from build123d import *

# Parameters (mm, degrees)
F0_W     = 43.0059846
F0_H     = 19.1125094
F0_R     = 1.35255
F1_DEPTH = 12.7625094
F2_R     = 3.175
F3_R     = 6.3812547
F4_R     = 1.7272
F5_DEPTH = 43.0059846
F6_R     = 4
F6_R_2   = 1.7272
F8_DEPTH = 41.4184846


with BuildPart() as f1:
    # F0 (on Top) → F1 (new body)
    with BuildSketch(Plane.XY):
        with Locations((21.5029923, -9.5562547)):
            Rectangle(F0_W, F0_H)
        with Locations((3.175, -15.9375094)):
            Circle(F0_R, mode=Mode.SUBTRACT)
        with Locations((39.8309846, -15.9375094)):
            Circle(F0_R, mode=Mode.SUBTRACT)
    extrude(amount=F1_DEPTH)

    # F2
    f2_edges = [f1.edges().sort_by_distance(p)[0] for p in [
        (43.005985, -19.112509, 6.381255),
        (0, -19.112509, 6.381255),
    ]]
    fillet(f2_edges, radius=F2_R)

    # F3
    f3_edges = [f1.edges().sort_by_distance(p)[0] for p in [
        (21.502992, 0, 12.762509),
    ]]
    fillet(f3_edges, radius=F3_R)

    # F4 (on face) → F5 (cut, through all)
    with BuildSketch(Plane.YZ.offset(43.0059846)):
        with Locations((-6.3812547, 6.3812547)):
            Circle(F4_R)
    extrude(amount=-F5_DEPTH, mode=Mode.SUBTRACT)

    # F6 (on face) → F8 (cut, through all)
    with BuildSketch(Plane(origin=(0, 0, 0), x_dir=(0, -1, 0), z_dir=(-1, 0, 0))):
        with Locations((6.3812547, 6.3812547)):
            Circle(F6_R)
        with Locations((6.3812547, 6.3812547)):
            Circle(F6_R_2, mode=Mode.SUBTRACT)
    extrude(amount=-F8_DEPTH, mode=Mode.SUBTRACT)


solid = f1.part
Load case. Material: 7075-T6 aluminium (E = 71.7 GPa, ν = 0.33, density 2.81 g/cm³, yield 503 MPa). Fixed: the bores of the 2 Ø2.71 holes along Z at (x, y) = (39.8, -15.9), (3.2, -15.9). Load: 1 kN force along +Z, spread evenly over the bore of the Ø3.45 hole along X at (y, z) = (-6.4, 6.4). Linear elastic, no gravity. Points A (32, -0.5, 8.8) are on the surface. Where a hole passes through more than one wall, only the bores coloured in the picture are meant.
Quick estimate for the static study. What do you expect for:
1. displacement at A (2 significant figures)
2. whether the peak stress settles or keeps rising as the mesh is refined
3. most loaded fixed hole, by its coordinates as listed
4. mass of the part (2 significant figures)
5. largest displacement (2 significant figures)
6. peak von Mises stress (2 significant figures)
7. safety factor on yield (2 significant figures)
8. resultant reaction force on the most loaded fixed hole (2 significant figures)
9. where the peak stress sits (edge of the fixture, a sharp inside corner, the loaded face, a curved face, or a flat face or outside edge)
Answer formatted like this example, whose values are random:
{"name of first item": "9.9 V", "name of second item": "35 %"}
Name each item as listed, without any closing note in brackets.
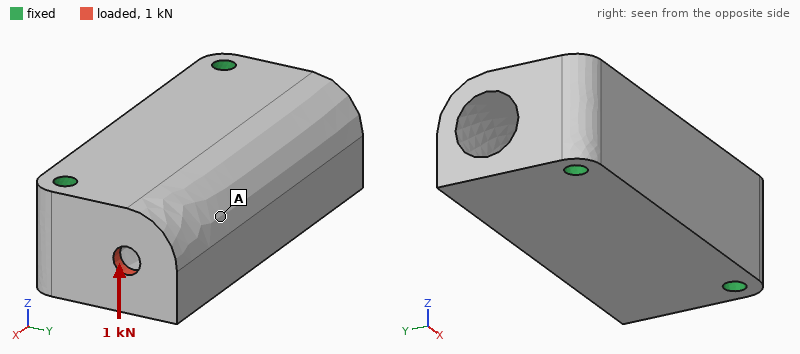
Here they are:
{"displacement at A": "7.6 µm", "whether the peak stress settles or keeps rising as the mesh is refined": "settles", "most loaded fixed hole, by its coordinates as listed": "(39.8, -15.9)", "mass of the part": "22 g", "largest displacement": "15 µm", "peak von Mises stress": "130 MPa", "safety factor on yield": "3.8", "resultant reaction force on the most loaded fixed hole": "1.0 kN", "where the peak stress sits": "the loaded face"}
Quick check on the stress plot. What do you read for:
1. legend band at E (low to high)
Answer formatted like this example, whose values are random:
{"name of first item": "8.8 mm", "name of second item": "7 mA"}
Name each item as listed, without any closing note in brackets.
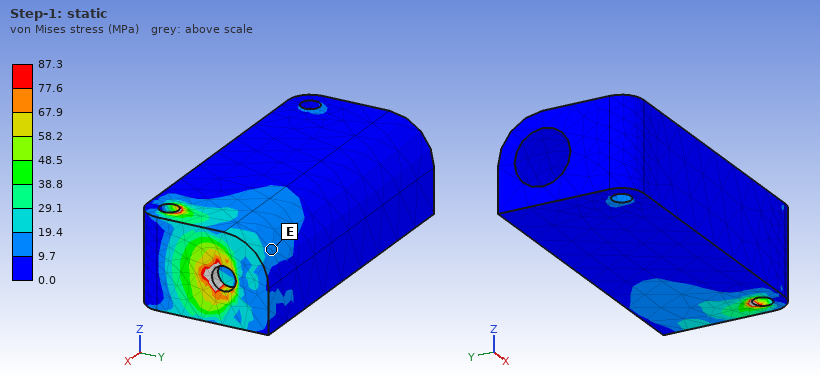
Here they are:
{"legend band at E": "9.7 to 19.4 MPa"}
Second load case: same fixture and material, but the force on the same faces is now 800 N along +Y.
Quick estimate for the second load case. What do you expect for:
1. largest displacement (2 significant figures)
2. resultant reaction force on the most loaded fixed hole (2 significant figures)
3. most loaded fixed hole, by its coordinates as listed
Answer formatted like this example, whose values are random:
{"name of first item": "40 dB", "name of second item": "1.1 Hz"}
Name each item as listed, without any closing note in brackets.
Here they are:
{"largest displacement": "5.7 µm", "resultant reaction force on the most loaded fixed hole": "850 N", "most loaded fixed hole, by its coordinates as listed": "(39.8, -15.9)"}
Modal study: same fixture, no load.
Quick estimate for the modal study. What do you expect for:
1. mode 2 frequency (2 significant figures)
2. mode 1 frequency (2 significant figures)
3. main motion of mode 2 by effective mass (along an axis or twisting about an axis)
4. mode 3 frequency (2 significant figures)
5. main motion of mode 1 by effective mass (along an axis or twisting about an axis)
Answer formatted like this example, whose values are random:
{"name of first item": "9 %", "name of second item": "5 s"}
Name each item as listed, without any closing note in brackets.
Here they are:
{"mode 2 frequency": "27 kHz", "mode 1 frequency": "17 kHz", "main motion of mode 2 by effective mass": "along Y", "mode 3 frequency": "30 kHz", "main motion of mode 1 by effective mass": "along Z"}
